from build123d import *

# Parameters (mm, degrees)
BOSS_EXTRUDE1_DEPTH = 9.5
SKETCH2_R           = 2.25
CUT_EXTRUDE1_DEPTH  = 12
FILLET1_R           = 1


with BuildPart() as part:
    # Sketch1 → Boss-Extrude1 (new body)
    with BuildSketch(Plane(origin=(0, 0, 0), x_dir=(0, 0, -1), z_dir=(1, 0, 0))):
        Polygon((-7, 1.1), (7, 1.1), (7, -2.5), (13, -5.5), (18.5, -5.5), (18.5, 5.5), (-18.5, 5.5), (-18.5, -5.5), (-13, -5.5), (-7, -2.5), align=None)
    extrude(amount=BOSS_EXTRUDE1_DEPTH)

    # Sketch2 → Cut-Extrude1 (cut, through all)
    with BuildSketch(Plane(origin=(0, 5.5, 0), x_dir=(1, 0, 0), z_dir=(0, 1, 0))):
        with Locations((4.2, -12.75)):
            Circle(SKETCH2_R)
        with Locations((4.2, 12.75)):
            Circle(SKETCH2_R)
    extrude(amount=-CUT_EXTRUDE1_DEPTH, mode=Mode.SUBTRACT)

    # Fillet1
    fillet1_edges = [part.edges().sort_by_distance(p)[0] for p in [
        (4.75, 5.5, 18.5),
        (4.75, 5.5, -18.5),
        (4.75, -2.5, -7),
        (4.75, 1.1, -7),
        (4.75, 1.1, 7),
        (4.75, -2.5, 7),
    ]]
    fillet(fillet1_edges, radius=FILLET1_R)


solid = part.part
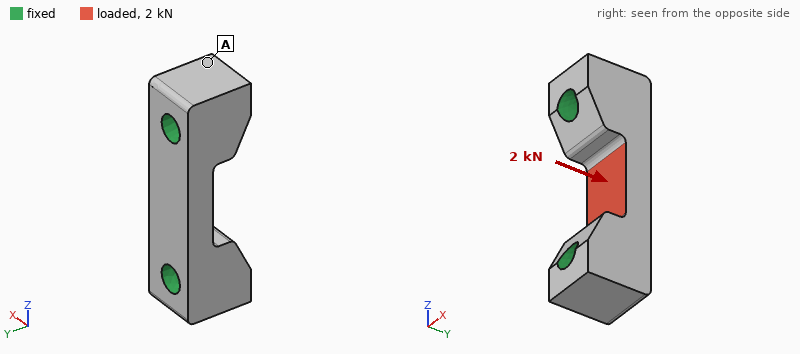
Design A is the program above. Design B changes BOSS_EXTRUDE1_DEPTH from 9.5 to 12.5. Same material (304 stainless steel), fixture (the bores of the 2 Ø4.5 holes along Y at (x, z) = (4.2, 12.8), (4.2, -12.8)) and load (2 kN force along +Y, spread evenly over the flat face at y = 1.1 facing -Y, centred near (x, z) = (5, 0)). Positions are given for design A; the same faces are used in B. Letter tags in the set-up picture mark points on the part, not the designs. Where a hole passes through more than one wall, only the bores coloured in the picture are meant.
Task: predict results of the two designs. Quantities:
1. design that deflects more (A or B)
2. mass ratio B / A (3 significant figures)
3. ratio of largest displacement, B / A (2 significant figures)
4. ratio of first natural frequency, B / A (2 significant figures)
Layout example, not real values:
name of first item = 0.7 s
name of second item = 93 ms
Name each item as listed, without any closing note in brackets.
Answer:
design that deflects more = A
mass ratio B / A = 1.36
ratio of largest displacement, B / A = 0.89
ratio of first natural frequency, B / A = 0.91
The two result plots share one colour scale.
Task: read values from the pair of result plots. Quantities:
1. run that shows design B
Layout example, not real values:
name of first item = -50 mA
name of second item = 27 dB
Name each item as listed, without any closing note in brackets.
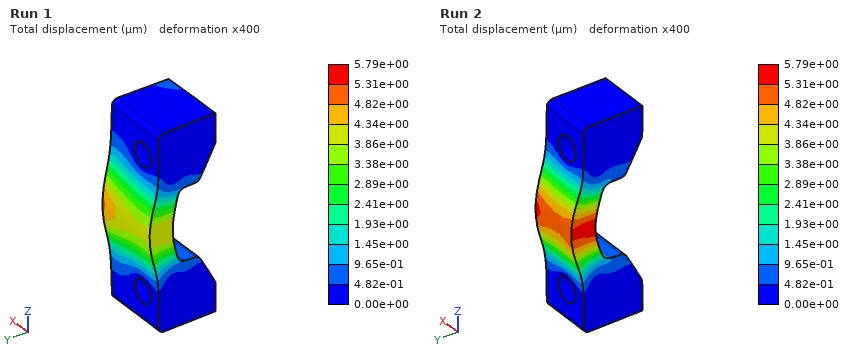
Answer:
run that shows design B = Run 1
